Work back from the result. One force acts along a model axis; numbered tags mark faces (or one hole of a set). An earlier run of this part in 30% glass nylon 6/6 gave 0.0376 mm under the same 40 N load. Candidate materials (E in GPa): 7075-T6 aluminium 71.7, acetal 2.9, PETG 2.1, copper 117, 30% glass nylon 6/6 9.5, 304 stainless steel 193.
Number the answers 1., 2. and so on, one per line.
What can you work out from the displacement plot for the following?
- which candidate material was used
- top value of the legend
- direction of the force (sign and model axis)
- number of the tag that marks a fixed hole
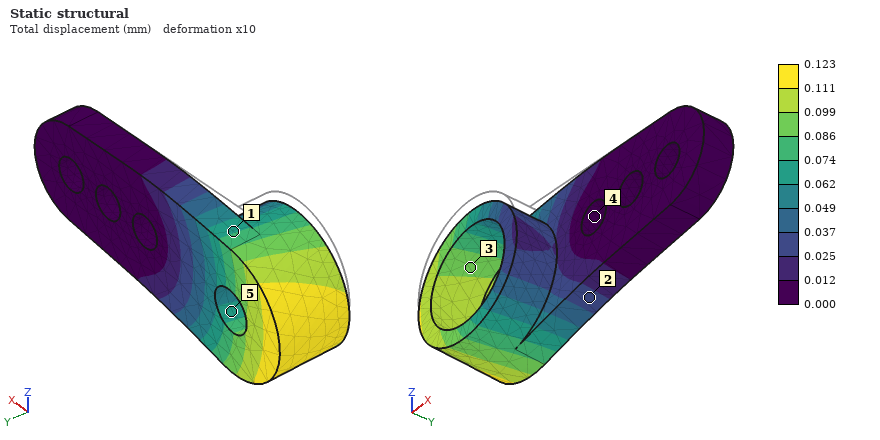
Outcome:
1. acetal
2. 0.123 mm
3. -Z
4. 4
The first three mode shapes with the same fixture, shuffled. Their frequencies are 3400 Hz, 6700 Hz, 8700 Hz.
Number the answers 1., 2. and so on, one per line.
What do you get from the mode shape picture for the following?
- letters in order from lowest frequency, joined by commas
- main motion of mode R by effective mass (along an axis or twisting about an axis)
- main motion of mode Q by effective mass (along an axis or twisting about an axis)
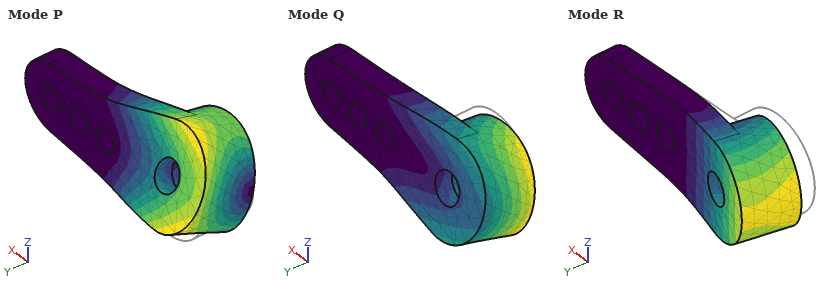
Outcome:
1. R, Q, P
2. along Y
3. along Z
